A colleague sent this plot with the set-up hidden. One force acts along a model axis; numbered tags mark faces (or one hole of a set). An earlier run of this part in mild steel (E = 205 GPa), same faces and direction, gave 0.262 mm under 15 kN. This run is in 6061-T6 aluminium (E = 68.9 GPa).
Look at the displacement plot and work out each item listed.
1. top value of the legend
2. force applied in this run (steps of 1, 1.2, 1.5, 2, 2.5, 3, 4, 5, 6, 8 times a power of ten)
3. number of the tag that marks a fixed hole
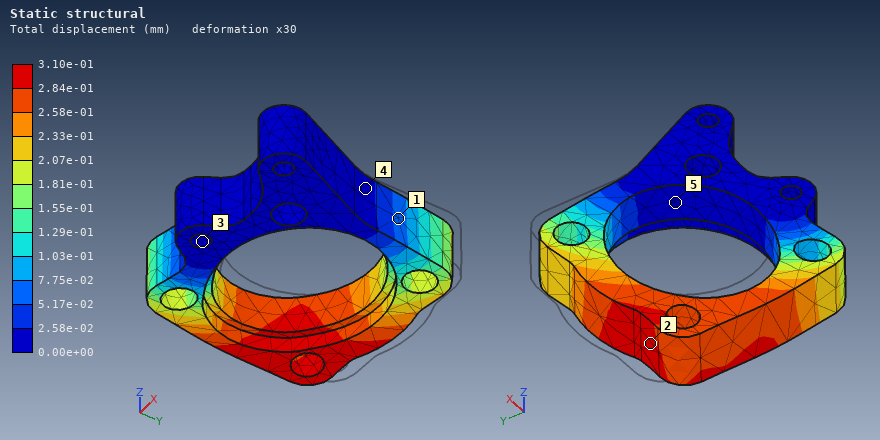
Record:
3.10e-01 mm
6 kN
3
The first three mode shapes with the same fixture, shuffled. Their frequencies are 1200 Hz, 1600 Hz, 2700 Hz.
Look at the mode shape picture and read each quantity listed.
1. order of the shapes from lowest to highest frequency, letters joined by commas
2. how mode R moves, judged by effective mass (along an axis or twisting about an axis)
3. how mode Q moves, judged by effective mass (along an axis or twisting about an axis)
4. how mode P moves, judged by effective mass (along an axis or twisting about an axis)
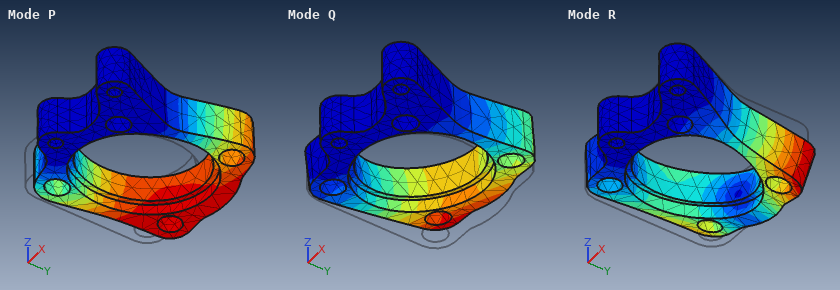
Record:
Q, P, R
twisting about Y
along Z
along X
